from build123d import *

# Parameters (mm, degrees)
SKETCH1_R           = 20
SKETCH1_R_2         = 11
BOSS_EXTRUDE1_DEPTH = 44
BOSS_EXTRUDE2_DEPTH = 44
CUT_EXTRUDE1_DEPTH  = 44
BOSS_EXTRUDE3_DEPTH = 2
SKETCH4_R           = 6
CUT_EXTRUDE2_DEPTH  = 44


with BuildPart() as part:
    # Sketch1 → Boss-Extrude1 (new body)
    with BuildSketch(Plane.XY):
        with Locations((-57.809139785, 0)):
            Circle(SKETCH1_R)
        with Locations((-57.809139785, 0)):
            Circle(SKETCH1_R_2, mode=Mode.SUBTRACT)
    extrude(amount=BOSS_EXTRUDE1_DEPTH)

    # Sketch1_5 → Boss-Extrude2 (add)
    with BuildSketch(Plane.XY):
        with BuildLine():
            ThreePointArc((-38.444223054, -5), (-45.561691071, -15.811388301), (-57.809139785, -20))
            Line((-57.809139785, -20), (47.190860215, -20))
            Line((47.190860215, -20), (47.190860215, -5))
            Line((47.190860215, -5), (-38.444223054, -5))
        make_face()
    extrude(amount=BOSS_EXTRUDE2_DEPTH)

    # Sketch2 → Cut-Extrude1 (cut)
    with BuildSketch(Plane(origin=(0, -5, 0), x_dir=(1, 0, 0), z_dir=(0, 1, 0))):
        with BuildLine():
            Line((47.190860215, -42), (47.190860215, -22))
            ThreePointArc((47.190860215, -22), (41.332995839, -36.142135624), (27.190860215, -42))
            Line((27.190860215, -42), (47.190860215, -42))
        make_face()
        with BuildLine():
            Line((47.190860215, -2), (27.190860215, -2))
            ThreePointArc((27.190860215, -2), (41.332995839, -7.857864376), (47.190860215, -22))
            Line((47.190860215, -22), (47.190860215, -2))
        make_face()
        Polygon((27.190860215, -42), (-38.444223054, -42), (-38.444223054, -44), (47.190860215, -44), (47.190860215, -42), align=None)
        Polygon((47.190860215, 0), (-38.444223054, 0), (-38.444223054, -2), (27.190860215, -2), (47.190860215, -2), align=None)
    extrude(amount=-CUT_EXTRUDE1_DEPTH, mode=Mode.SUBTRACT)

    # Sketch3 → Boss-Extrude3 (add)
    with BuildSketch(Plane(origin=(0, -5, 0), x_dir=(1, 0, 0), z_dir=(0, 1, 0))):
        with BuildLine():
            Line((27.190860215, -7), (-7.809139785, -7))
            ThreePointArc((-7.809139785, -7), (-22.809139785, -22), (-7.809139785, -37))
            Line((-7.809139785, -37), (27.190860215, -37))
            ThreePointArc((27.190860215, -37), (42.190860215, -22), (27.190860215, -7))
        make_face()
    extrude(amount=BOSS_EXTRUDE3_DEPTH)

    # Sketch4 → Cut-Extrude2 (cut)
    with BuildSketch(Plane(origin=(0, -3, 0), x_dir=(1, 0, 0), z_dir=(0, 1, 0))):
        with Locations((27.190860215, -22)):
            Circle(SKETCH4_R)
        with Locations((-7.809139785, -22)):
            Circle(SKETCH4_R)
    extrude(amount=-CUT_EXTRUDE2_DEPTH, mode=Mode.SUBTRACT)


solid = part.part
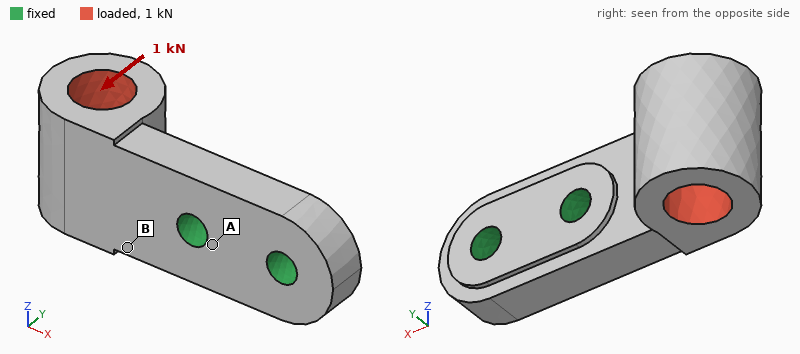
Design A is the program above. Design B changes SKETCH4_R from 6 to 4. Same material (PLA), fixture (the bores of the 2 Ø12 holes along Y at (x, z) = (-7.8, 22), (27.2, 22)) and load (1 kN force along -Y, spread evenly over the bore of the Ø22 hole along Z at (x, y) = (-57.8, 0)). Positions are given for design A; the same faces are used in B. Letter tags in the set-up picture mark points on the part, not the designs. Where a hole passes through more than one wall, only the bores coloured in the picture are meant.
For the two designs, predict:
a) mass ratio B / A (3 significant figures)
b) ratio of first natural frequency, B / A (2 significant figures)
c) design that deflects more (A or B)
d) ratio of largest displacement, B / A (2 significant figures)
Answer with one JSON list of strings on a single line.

["1.02", "0.94", "B", "1.1"]
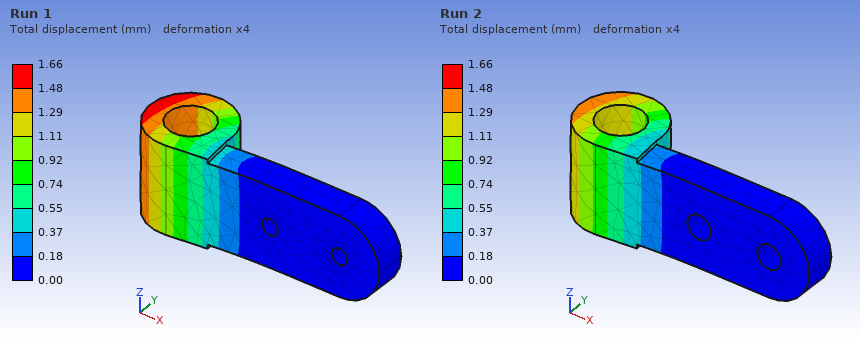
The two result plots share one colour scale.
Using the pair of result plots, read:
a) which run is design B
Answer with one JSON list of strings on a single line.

["Run 1"]
